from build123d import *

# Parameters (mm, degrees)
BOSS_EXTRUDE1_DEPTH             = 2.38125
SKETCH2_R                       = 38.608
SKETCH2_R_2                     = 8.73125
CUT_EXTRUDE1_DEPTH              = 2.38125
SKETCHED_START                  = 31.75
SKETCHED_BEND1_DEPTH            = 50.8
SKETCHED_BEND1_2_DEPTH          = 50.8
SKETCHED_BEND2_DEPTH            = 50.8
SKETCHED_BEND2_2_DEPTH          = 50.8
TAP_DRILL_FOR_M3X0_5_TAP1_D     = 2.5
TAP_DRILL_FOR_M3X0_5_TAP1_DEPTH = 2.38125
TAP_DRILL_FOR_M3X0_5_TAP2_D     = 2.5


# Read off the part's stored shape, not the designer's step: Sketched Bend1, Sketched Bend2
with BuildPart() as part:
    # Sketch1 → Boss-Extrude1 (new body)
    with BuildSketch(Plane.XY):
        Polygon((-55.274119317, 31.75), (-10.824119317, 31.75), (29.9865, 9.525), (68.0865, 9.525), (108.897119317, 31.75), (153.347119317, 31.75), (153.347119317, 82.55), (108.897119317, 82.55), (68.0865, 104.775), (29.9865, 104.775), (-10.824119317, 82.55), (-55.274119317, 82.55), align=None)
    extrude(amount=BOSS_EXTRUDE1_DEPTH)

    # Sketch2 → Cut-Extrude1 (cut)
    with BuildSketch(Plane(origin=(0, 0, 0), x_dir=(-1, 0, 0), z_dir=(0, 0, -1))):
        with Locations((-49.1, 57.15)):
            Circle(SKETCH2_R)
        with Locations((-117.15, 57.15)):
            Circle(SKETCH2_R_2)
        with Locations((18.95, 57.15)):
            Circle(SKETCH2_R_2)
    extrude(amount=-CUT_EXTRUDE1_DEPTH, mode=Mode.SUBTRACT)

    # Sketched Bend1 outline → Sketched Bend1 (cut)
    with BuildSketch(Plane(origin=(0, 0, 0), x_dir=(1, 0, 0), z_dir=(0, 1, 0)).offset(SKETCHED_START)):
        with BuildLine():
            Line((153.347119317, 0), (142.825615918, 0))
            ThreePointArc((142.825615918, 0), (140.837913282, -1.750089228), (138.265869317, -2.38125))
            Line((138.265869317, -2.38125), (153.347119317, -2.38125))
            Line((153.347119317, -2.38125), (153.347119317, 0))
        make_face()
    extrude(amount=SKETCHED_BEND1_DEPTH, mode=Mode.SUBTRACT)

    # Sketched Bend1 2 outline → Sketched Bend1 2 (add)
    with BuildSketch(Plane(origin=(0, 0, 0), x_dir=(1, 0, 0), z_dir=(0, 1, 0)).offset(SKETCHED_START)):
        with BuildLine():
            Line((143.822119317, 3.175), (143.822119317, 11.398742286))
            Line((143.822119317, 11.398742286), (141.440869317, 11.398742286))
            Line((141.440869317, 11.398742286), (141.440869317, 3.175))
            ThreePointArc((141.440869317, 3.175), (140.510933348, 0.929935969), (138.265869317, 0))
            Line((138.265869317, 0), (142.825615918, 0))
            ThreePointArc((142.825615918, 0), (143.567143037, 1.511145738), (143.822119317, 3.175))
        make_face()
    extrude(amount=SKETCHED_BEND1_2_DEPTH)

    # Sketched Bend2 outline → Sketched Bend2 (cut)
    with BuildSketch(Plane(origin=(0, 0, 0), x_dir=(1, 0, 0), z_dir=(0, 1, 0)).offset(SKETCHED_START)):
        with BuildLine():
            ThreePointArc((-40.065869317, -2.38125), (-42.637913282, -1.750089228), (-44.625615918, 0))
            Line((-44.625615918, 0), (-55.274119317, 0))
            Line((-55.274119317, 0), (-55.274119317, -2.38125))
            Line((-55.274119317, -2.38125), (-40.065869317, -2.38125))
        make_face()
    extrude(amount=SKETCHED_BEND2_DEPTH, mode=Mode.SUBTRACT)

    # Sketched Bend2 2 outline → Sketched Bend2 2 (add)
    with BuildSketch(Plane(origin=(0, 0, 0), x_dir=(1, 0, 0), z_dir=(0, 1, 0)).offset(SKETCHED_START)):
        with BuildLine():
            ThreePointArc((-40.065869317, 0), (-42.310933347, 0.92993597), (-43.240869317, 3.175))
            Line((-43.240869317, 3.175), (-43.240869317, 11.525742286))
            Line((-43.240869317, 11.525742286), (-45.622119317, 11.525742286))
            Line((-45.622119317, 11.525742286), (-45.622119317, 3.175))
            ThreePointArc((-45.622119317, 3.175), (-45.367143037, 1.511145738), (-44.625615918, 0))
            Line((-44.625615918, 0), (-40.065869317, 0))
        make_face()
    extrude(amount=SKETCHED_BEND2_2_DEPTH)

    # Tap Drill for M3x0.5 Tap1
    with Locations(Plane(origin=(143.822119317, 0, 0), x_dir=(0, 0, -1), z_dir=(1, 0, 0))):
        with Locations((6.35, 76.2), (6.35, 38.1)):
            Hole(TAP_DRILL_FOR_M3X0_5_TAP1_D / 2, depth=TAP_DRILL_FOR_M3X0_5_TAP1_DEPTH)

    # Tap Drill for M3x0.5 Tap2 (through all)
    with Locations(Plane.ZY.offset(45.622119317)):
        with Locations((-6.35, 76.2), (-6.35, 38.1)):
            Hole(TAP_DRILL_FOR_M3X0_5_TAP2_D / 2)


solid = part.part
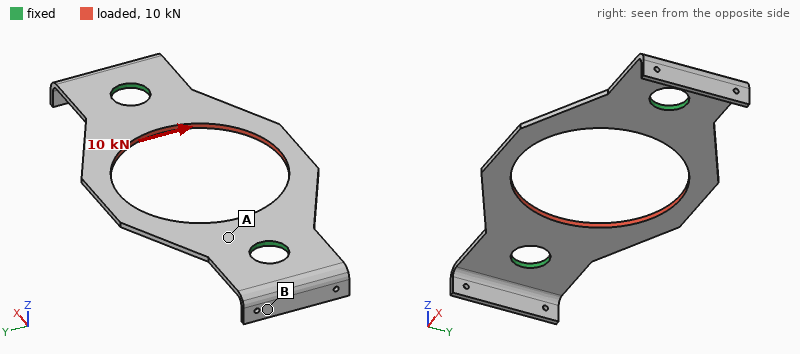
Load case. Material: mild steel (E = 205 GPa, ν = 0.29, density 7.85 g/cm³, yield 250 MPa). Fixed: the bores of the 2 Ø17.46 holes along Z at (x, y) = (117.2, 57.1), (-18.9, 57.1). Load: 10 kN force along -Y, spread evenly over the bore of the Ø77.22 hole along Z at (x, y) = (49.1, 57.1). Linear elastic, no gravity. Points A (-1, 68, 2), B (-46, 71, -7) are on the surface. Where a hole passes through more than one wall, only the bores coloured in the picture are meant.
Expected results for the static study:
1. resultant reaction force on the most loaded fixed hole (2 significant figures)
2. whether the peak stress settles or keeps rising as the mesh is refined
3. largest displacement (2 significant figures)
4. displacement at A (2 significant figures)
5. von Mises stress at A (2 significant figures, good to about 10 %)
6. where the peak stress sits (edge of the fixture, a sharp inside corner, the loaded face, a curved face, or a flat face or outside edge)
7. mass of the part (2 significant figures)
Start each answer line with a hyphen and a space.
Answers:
- 5.0 kN
- keeps rising
- 44 µm
- 9.9 µm
- 74 MPa
- edge of the fixture
- 170 g
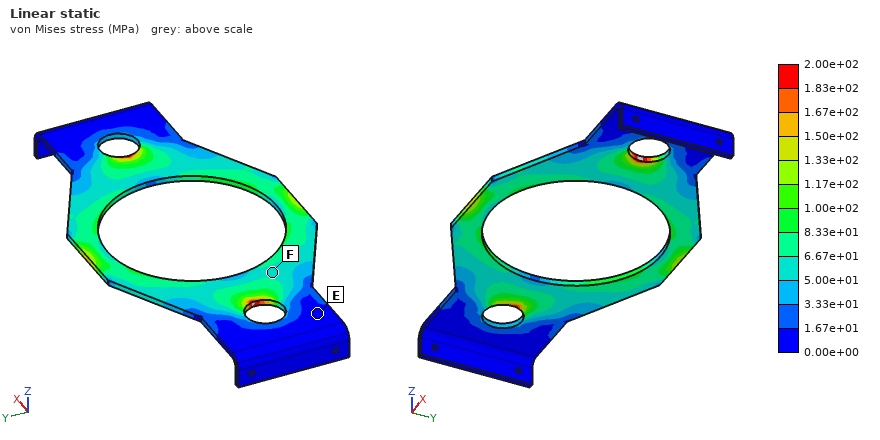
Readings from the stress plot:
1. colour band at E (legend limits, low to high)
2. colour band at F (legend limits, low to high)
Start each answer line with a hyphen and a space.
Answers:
- 0.00e+00 to 1.67e+01 MPa
- 5.00e+01 to 6.67e+01 MPa
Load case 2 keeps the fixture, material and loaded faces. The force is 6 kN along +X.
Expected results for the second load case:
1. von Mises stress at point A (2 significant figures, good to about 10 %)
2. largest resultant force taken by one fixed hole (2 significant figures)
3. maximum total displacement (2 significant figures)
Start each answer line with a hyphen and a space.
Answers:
- 22 MPa
- 3.0 kN
- 18 µm
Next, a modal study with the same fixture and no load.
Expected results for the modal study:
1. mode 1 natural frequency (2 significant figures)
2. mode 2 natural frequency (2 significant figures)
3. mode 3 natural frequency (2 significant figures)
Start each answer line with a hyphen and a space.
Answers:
- 680 Hz
- 700 Hz
- 1600 Hz
